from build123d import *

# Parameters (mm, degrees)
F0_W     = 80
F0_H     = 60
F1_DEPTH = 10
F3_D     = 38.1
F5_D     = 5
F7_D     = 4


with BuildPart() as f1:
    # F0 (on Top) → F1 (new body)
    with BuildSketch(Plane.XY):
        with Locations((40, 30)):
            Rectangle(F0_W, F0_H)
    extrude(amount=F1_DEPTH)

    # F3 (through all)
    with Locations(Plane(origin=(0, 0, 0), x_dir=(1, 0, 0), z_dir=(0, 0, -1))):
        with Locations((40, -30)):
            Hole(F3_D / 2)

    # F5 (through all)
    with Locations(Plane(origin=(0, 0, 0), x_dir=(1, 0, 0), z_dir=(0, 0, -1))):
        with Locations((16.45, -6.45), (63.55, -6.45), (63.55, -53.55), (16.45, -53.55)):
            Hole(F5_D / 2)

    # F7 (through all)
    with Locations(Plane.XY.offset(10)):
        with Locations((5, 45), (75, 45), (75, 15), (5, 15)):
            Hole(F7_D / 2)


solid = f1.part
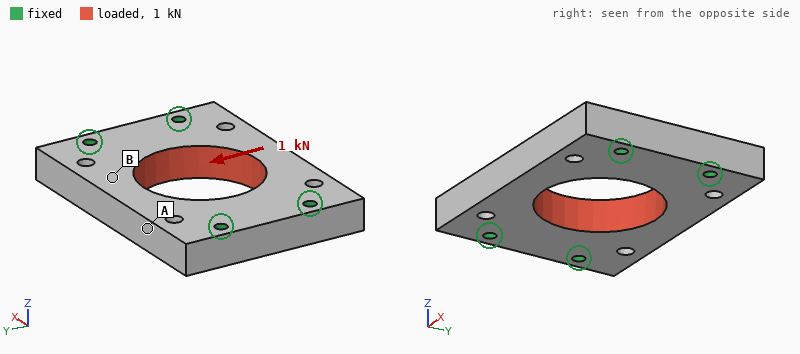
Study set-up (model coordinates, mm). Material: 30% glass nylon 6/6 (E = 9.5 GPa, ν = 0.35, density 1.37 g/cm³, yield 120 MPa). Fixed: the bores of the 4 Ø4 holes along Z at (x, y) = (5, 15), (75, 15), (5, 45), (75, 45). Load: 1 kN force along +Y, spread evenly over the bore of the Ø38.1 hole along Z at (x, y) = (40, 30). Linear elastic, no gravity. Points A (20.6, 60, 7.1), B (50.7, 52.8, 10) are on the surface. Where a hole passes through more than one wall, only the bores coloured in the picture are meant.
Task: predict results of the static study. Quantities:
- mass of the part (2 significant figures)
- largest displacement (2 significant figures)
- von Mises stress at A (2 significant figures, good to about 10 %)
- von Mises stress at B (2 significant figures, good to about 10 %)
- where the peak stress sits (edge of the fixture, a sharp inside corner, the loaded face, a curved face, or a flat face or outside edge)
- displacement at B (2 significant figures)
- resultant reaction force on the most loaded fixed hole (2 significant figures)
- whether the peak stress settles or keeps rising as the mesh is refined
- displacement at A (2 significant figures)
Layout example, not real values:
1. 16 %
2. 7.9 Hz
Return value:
1. 48 g
2. 14 µm
3. 0.83 MPa
4. 1.7 MPa
5. edge of the fixture
6. 11 µm
7. 260 N
8. keeps rising
9. 8.2 µm
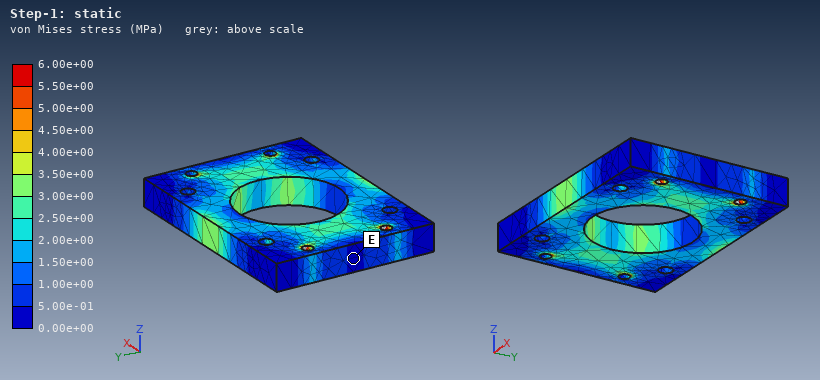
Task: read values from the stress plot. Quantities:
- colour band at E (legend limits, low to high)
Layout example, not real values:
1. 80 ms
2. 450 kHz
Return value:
1. 0.00e+00 to 5.00e-01 MPa
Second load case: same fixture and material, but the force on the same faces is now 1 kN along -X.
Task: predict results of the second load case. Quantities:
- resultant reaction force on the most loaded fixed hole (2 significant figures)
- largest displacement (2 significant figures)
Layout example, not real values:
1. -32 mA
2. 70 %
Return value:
1. 250 N
2. 5.0 µm
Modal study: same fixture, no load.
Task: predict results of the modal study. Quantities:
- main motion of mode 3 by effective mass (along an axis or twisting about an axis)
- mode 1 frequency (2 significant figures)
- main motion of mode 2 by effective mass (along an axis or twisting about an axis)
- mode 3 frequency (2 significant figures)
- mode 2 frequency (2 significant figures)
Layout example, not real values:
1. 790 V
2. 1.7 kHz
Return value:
1. twisting about Y
2. 4600 Hz
3. twisting about X
4. 9600 Hz
5. 4800 Hz
